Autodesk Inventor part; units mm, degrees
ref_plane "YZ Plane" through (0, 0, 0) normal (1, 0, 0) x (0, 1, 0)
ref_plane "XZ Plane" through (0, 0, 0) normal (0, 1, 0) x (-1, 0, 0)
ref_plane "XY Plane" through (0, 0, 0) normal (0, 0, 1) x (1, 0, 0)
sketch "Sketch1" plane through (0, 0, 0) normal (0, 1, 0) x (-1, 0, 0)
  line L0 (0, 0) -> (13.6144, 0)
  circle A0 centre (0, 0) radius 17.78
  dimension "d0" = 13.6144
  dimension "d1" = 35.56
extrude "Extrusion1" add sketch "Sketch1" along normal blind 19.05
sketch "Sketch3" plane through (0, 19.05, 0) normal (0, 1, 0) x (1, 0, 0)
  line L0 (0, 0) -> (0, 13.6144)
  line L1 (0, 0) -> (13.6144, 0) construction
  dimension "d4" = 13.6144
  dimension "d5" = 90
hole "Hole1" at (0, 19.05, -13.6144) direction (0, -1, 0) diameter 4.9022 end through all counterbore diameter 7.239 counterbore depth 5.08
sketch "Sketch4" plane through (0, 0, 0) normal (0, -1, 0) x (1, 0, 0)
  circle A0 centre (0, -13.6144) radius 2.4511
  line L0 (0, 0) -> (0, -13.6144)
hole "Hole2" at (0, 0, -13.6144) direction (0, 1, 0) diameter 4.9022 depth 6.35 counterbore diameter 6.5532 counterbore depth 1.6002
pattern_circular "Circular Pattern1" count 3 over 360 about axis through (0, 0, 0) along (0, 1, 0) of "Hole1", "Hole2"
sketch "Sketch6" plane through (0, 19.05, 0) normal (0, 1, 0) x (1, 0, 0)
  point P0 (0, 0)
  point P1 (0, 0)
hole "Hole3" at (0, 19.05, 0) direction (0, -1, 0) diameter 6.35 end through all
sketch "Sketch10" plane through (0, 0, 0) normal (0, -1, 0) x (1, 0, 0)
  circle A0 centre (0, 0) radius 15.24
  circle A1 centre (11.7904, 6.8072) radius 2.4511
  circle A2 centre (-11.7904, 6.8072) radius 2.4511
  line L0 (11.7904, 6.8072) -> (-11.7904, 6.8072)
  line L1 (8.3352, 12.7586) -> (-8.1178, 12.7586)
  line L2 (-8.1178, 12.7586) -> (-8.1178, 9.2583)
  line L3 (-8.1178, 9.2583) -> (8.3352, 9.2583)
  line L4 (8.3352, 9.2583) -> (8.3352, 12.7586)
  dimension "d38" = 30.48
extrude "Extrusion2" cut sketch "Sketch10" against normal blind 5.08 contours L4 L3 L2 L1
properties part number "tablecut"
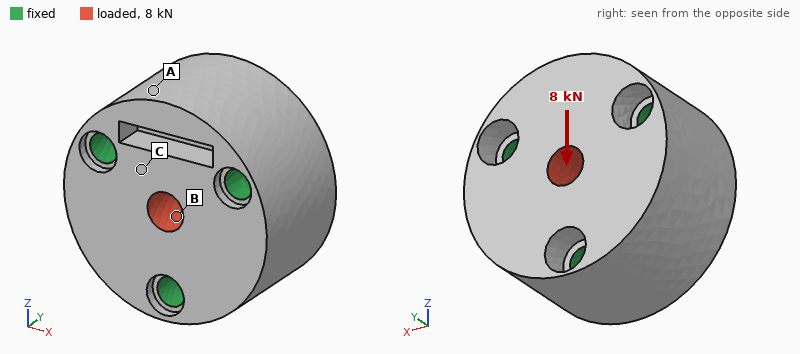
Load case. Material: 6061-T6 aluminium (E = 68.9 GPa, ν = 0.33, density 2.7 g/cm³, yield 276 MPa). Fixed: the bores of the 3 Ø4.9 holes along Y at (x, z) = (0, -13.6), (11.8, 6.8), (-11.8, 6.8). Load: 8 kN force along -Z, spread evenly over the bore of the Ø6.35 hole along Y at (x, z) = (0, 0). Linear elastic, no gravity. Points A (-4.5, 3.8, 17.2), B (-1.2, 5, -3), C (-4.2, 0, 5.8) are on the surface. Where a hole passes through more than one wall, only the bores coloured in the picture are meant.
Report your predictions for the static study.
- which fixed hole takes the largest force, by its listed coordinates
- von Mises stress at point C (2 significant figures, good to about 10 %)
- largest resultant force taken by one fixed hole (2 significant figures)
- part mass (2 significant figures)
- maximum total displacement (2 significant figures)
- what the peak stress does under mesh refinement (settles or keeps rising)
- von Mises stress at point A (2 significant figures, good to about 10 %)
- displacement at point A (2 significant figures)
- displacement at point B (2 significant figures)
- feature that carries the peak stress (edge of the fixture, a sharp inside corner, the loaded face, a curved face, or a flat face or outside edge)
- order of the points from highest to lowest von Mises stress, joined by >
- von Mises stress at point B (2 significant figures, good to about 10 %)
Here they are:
(0, -13.6)
19 MPa
3.0 kN
45 g
5.3 µm
keeps rising
7.2 MPa
1.7 µm
2.8 µm
edge of the fixture
B > C > A
26 MPa
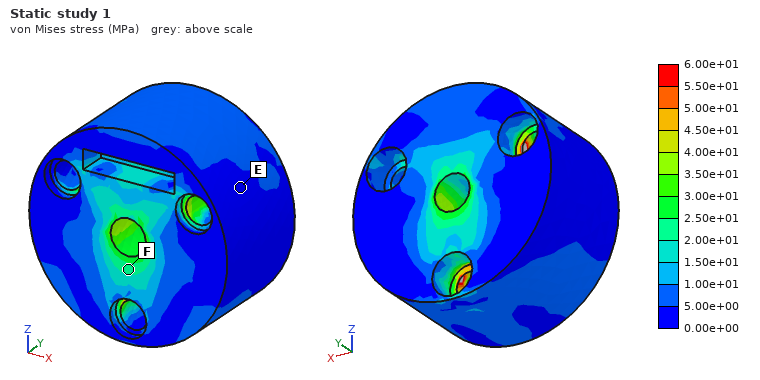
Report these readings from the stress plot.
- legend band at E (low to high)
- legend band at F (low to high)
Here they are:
0.00e+00 to 5.00e+00 MPa
2.00e+01 to 2.50e+01 MPa
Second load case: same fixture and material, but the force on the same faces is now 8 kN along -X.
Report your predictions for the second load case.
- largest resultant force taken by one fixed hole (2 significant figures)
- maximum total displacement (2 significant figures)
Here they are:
2.8 kN
4.9 µm
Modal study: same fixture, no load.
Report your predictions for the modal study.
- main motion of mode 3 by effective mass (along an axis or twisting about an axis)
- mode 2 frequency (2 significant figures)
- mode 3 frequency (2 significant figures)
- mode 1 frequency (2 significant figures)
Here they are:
along Y
39 kHz
45 kHz
38 kHz
